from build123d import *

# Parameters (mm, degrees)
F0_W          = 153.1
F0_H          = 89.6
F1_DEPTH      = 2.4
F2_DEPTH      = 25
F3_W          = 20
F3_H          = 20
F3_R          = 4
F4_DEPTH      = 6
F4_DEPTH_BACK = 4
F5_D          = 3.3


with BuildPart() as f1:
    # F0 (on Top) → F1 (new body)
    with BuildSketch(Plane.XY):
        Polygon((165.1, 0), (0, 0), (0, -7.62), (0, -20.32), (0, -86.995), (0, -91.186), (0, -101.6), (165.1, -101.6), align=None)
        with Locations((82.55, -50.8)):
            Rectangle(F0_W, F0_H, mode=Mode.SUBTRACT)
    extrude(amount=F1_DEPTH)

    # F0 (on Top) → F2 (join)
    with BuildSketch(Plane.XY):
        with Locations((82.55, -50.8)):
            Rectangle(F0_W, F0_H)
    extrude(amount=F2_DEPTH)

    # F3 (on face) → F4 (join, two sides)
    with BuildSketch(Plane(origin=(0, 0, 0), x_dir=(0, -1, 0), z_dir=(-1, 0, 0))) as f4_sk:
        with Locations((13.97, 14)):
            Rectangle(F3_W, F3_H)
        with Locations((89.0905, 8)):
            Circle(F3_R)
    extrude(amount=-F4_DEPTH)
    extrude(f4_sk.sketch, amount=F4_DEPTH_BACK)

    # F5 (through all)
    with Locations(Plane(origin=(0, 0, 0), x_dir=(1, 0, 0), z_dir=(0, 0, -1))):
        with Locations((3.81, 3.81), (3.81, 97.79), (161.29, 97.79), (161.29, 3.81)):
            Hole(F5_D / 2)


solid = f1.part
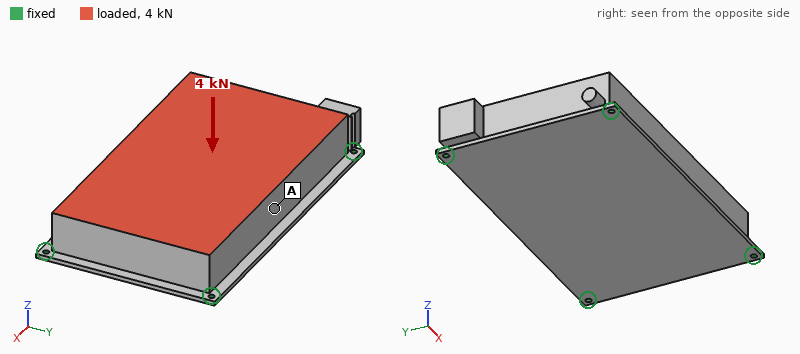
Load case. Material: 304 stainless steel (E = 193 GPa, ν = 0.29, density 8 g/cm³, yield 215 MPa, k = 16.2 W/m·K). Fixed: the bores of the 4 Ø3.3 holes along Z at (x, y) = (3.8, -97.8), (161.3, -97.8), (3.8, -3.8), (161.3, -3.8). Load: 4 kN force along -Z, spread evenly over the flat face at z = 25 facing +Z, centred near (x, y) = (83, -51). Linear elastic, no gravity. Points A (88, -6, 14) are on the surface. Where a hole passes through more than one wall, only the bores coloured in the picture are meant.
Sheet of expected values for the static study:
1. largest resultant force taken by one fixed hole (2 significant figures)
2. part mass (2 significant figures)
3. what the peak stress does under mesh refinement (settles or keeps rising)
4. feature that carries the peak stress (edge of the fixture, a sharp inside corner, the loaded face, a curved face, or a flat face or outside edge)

1.4 kN
2.8 kg
keeps rising
edge of the fixture
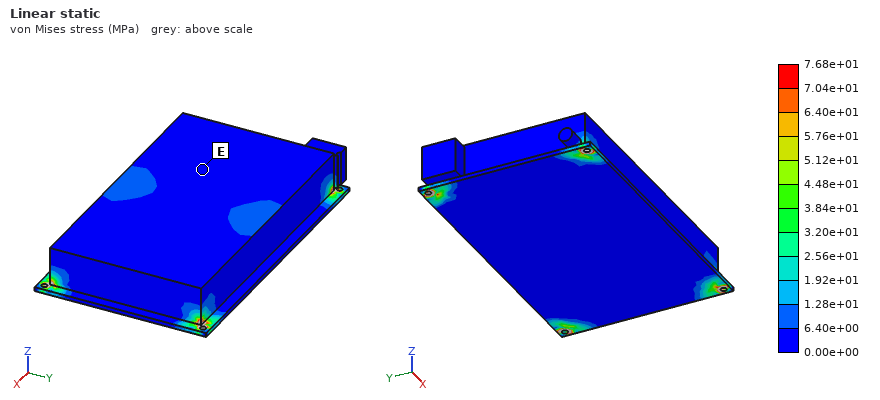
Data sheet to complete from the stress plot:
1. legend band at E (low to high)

0.00e+00 to 6.40e+00 MPa
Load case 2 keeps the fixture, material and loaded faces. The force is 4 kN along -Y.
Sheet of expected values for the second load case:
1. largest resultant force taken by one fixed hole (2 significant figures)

1.3 kN
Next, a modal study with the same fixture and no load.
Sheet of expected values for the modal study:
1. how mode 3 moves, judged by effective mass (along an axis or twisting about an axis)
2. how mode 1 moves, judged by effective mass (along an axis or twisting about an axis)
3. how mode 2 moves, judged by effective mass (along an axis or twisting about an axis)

twisting about Y
along Z
along Y
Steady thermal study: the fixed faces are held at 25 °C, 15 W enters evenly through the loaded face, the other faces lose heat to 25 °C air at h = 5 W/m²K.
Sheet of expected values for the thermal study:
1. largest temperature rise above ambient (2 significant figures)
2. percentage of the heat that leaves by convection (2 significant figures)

42 K
41 %
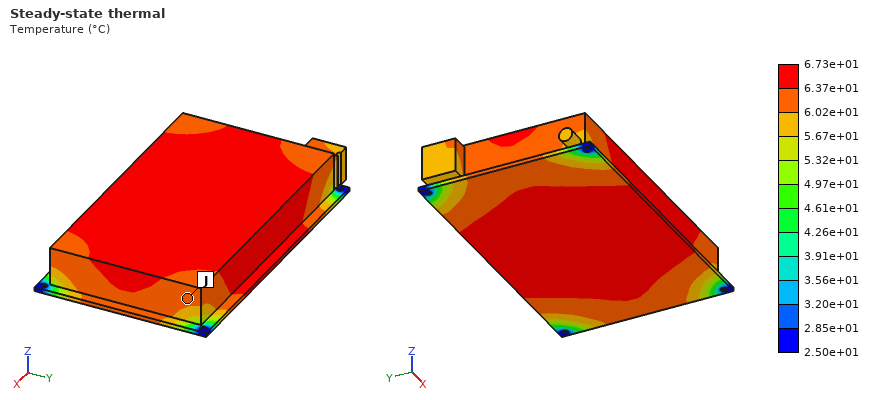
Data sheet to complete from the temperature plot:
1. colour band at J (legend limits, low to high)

6.02e+01 to 6.37e+01 °C
